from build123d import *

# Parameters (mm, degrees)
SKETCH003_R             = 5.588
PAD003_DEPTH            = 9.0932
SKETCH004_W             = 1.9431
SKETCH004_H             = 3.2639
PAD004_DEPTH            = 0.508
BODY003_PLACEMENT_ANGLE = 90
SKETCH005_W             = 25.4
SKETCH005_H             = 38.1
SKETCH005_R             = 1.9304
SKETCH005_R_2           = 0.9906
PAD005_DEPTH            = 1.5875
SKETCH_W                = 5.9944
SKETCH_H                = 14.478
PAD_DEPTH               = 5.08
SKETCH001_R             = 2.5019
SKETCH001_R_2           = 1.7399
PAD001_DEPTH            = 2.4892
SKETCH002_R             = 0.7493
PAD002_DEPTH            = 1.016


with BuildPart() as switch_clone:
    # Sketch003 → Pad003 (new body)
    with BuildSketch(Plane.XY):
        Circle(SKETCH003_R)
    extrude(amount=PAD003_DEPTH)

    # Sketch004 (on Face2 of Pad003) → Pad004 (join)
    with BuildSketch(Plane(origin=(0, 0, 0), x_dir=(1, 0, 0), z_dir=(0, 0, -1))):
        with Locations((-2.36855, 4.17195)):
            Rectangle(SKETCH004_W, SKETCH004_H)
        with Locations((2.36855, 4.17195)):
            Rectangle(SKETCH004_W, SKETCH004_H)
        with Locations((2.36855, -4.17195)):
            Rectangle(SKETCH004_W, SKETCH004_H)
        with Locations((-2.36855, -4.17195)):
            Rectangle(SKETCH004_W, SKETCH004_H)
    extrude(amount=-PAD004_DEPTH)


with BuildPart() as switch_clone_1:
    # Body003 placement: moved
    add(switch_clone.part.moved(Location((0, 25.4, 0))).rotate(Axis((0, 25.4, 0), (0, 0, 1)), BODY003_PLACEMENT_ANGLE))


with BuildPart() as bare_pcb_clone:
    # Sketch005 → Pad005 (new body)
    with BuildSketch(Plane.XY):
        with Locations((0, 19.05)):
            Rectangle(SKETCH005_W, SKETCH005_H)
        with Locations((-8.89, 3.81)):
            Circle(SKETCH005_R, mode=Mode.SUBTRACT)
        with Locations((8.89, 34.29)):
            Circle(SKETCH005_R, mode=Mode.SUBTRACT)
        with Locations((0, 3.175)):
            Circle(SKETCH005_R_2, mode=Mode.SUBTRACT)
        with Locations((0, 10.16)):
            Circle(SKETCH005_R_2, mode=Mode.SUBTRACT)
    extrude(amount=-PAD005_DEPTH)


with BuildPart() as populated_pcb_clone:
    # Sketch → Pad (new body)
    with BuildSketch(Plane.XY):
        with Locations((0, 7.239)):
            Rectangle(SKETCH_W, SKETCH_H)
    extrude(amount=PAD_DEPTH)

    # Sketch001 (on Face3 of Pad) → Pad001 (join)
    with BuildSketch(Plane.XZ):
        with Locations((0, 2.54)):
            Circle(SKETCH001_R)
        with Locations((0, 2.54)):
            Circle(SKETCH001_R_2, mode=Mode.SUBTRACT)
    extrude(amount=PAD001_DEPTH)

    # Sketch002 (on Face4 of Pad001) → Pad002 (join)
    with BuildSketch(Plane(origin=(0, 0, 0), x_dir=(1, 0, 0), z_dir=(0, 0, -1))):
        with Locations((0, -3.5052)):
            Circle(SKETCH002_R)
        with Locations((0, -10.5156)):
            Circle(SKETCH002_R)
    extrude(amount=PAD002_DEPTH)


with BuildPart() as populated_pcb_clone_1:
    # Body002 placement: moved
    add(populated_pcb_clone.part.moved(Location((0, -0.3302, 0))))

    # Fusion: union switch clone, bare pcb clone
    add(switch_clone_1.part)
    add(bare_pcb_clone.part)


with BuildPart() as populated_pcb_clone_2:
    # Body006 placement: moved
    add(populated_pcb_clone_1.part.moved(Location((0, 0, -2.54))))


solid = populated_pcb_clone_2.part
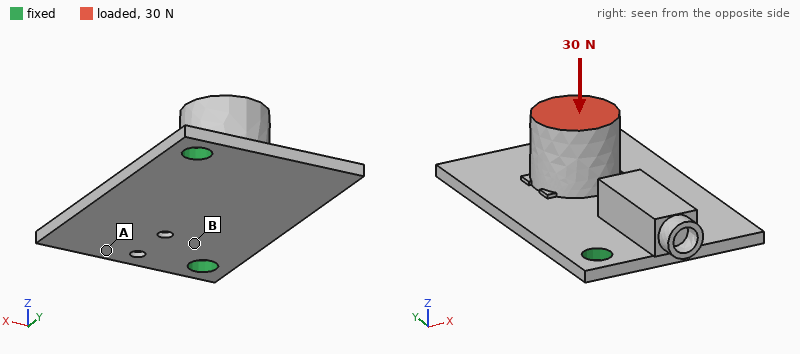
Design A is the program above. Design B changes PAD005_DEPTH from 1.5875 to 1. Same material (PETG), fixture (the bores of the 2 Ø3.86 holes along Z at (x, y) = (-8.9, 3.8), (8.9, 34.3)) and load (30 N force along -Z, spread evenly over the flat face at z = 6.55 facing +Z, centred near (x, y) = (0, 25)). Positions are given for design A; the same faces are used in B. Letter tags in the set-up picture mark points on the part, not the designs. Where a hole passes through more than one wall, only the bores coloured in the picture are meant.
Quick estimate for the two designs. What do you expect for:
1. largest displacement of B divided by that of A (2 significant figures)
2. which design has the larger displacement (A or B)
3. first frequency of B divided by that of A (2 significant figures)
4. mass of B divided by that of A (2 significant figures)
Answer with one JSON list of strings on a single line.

["3.3", "B", "0.62", "0.81"]
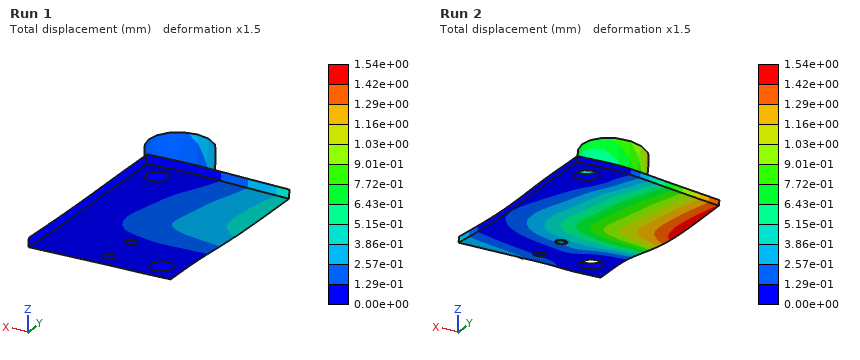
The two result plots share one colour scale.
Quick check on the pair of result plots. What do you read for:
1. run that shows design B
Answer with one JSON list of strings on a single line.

["Run 2"]
